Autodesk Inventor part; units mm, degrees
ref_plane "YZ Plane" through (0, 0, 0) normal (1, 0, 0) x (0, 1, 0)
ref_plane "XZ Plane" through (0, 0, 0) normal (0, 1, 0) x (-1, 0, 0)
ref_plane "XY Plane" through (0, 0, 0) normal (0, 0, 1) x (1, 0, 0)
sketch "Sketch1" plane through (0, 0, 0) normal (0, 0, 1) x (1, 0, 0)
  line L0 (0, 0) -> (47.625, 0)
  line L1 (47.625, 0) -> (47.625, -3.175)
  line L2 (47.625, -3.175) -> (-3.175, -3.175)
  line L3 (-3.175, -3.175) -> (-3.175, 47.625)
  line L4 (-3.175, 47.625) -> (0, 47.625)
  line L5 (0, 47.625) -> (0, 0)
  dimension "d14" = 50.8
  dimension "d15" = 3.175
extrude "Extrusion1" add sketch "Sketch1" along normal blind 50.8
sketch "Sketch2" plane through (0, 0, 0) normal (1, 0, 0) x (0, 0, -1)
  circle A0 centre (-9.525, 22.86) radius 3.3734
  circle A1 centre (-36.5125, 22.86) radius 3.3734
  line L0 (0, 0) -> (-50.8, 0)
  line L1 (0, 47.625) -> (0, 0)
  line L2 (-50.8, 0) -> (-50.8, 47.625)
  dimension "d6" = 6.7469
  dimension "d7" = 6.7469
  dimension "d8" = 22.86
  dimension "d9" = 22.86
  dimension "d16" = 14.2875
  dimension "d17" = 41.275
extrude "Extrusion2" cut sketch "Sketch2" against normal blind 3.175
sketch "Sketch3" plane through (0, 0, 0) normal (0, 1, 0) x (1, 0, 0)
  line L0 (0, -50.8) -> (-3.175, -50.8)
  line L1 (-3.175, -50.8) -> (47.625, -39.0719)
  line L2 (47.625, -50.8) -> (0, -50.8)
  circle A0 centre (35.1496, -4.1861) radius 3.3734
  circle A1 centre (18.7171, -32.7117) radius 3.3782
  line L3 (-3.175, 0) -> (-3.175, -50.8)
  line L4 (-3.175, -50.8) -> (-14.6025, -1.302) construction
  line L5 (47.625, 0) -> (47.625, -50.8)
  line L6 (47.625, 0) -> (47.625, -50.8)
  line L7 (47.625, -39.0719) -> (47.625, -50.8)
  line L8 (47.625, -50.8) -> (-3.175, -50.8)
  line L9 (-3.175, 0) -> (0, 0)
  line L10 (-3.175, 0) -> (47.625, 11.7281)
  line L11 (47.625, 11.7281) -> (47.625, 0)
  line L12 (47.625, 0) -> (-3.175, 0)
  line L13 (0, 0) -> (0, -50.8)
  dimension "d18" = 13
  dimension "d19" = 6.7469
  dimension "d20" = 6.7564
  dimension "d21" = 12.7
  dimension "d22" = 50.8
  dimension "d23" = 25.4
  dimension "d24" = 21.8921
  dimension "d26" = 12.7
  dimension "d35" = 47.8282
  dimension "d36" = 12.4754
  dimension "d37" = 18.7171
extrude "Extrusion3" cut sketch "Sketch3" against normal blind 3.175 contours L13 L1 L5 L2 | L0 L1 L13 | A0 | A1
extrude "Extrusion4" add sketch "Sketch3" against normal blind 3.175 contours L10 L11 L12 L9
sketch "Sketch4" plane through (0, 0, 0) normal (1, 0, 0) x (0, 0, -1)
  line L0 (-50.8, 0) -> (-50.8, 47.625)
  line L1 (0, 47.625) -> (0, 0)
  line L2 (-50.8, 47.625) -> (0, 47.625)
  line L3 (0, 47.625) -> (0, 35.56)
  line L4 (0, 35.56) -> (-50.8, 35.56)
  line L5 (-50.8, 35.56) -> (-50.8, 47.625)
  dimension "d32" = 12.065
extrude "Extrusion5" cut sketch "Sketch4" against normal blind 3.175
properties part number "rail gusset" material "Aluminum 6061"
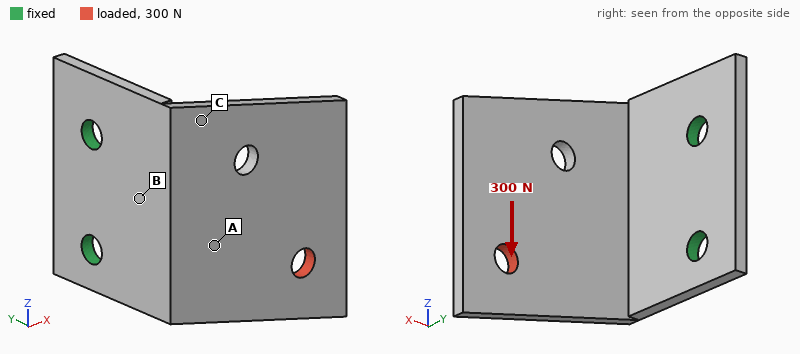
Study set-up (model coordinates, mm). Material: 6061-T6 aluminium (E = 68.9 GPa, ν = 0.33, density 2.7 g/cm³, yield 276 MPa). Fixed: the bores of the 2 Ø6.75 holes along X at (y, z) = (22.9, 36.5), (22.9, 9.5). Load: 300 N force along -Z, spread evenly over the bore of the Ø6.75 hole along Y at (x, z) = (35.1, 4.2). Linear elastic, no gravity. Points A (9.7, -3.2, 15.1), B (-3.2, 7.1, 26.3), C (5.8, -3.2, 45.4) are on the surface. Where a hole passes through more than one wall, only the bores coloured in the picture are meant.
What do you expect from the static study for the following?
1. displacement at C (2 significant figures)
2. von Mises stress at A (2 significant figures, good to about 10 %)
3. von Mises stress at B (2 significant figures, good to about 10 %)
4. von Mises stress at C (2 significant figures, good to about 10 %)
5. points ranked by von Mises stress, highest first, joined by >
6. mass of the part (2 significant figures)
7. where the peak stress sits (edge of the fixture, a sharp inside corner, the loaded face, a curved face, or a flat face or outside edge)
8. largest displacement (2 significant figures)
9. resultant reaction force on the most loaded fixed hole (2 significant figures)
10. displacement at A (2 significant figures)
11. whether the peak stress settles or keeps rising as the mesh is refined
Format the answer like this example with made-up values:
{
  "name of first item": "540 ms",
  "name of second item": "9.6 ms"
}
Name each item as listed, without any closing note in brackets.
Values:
{
  "displacement at C": "0.17 mm",
  "von Mises stress at A": "15 MPa",
  "von Mises stress at B": "52 MPa",
  "von Mises stress at C": "32 MPa",
  "points ranked by von Mises stress, highest first, joined by >": "B > C > A",
  "mass of the part": "36 g",
  "where the peak stress sits": "edge of the fixture",
  "largest displacement": "0.47 mm",
  "resultant reaction force on the most loaded fixed hole": "420 N",
  "displacement at A": "0.11 mm",
  "whether the peak stress settles or keeps rising as the mesh is refined": "keeps rising"
}
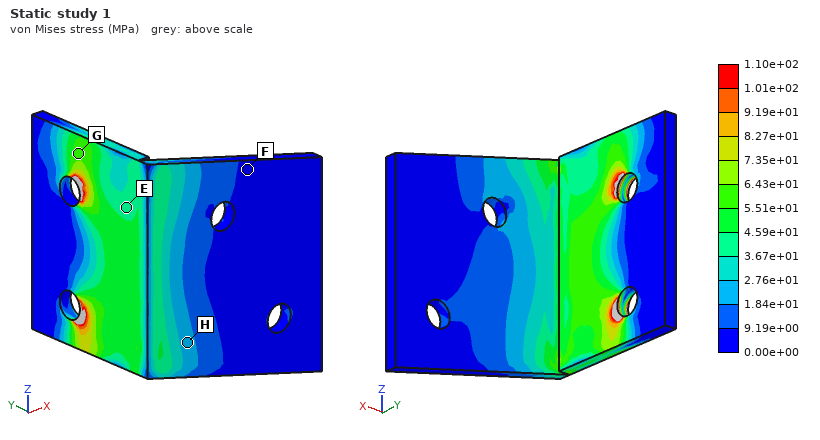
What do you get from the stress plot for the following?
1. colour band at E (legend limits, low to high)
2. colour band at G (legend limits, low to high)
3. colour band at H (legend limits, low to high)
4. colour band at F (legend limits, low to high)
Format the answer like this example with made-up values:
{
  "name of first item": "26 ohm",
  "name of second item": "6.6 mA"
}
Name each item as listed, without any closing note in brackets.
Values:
{
  "colour band at E": "3.67e+01 to 4.59e+01 MPa",
  "colour band at G": "5.51e+01 to 6.43e+01 MPa",
  "colour band at H": "1.84e+01 to 2.76e+01 MPa",
  "colour band at F": "0.00e+00 to 9.19e+00 MPa"
}
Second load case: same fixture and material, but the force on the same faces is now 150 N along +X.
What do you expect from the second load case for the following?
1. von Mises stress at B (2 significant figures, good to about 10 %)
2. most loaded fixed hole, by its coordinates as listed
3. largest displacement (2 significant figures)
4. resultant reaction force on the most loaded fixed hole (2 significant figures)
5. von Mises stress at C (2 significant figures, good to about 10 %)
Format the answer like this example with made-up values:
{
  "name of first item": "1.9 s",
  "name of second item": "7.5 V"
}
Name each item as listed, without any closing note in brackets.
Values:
{
  "von Mises stress at B": "20 MPa",
  "most loaded fixed hole, by its coordinates as listed": "(22.9, 9.5)",
  "largest displacement": "0.29 mm",
  "resultant reaction force on the most loaded fixed hole": "160 N",
  "von Mises stress at C": "9.7 MPa"
}
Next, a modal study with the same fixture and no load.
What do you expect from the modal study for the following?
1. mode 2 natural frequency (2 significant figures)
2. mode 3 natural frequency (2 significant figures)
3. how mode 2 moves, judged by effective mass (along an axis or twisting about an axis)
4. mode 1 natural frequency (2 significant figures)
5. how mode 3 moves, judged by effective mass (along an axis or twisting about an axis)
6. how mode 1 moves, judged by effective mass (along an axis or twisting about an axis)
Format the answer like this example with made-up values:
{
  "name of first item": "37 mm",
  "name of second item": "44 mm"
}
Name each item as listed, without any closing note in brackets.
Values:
{
  "mode 2 natural frequency": "1300 Hz",
  "mode 3 natural frequency": "2100 Hz",
  "how mode 2 moves, judged by effective mass": "along Z",
  "mode 1 natural frequency": "630 Hz",
  "how mode 3 moves, judged by effective mass": "along X",
  "how mode 1 moves, judged by effective mass": "along Y"
}
